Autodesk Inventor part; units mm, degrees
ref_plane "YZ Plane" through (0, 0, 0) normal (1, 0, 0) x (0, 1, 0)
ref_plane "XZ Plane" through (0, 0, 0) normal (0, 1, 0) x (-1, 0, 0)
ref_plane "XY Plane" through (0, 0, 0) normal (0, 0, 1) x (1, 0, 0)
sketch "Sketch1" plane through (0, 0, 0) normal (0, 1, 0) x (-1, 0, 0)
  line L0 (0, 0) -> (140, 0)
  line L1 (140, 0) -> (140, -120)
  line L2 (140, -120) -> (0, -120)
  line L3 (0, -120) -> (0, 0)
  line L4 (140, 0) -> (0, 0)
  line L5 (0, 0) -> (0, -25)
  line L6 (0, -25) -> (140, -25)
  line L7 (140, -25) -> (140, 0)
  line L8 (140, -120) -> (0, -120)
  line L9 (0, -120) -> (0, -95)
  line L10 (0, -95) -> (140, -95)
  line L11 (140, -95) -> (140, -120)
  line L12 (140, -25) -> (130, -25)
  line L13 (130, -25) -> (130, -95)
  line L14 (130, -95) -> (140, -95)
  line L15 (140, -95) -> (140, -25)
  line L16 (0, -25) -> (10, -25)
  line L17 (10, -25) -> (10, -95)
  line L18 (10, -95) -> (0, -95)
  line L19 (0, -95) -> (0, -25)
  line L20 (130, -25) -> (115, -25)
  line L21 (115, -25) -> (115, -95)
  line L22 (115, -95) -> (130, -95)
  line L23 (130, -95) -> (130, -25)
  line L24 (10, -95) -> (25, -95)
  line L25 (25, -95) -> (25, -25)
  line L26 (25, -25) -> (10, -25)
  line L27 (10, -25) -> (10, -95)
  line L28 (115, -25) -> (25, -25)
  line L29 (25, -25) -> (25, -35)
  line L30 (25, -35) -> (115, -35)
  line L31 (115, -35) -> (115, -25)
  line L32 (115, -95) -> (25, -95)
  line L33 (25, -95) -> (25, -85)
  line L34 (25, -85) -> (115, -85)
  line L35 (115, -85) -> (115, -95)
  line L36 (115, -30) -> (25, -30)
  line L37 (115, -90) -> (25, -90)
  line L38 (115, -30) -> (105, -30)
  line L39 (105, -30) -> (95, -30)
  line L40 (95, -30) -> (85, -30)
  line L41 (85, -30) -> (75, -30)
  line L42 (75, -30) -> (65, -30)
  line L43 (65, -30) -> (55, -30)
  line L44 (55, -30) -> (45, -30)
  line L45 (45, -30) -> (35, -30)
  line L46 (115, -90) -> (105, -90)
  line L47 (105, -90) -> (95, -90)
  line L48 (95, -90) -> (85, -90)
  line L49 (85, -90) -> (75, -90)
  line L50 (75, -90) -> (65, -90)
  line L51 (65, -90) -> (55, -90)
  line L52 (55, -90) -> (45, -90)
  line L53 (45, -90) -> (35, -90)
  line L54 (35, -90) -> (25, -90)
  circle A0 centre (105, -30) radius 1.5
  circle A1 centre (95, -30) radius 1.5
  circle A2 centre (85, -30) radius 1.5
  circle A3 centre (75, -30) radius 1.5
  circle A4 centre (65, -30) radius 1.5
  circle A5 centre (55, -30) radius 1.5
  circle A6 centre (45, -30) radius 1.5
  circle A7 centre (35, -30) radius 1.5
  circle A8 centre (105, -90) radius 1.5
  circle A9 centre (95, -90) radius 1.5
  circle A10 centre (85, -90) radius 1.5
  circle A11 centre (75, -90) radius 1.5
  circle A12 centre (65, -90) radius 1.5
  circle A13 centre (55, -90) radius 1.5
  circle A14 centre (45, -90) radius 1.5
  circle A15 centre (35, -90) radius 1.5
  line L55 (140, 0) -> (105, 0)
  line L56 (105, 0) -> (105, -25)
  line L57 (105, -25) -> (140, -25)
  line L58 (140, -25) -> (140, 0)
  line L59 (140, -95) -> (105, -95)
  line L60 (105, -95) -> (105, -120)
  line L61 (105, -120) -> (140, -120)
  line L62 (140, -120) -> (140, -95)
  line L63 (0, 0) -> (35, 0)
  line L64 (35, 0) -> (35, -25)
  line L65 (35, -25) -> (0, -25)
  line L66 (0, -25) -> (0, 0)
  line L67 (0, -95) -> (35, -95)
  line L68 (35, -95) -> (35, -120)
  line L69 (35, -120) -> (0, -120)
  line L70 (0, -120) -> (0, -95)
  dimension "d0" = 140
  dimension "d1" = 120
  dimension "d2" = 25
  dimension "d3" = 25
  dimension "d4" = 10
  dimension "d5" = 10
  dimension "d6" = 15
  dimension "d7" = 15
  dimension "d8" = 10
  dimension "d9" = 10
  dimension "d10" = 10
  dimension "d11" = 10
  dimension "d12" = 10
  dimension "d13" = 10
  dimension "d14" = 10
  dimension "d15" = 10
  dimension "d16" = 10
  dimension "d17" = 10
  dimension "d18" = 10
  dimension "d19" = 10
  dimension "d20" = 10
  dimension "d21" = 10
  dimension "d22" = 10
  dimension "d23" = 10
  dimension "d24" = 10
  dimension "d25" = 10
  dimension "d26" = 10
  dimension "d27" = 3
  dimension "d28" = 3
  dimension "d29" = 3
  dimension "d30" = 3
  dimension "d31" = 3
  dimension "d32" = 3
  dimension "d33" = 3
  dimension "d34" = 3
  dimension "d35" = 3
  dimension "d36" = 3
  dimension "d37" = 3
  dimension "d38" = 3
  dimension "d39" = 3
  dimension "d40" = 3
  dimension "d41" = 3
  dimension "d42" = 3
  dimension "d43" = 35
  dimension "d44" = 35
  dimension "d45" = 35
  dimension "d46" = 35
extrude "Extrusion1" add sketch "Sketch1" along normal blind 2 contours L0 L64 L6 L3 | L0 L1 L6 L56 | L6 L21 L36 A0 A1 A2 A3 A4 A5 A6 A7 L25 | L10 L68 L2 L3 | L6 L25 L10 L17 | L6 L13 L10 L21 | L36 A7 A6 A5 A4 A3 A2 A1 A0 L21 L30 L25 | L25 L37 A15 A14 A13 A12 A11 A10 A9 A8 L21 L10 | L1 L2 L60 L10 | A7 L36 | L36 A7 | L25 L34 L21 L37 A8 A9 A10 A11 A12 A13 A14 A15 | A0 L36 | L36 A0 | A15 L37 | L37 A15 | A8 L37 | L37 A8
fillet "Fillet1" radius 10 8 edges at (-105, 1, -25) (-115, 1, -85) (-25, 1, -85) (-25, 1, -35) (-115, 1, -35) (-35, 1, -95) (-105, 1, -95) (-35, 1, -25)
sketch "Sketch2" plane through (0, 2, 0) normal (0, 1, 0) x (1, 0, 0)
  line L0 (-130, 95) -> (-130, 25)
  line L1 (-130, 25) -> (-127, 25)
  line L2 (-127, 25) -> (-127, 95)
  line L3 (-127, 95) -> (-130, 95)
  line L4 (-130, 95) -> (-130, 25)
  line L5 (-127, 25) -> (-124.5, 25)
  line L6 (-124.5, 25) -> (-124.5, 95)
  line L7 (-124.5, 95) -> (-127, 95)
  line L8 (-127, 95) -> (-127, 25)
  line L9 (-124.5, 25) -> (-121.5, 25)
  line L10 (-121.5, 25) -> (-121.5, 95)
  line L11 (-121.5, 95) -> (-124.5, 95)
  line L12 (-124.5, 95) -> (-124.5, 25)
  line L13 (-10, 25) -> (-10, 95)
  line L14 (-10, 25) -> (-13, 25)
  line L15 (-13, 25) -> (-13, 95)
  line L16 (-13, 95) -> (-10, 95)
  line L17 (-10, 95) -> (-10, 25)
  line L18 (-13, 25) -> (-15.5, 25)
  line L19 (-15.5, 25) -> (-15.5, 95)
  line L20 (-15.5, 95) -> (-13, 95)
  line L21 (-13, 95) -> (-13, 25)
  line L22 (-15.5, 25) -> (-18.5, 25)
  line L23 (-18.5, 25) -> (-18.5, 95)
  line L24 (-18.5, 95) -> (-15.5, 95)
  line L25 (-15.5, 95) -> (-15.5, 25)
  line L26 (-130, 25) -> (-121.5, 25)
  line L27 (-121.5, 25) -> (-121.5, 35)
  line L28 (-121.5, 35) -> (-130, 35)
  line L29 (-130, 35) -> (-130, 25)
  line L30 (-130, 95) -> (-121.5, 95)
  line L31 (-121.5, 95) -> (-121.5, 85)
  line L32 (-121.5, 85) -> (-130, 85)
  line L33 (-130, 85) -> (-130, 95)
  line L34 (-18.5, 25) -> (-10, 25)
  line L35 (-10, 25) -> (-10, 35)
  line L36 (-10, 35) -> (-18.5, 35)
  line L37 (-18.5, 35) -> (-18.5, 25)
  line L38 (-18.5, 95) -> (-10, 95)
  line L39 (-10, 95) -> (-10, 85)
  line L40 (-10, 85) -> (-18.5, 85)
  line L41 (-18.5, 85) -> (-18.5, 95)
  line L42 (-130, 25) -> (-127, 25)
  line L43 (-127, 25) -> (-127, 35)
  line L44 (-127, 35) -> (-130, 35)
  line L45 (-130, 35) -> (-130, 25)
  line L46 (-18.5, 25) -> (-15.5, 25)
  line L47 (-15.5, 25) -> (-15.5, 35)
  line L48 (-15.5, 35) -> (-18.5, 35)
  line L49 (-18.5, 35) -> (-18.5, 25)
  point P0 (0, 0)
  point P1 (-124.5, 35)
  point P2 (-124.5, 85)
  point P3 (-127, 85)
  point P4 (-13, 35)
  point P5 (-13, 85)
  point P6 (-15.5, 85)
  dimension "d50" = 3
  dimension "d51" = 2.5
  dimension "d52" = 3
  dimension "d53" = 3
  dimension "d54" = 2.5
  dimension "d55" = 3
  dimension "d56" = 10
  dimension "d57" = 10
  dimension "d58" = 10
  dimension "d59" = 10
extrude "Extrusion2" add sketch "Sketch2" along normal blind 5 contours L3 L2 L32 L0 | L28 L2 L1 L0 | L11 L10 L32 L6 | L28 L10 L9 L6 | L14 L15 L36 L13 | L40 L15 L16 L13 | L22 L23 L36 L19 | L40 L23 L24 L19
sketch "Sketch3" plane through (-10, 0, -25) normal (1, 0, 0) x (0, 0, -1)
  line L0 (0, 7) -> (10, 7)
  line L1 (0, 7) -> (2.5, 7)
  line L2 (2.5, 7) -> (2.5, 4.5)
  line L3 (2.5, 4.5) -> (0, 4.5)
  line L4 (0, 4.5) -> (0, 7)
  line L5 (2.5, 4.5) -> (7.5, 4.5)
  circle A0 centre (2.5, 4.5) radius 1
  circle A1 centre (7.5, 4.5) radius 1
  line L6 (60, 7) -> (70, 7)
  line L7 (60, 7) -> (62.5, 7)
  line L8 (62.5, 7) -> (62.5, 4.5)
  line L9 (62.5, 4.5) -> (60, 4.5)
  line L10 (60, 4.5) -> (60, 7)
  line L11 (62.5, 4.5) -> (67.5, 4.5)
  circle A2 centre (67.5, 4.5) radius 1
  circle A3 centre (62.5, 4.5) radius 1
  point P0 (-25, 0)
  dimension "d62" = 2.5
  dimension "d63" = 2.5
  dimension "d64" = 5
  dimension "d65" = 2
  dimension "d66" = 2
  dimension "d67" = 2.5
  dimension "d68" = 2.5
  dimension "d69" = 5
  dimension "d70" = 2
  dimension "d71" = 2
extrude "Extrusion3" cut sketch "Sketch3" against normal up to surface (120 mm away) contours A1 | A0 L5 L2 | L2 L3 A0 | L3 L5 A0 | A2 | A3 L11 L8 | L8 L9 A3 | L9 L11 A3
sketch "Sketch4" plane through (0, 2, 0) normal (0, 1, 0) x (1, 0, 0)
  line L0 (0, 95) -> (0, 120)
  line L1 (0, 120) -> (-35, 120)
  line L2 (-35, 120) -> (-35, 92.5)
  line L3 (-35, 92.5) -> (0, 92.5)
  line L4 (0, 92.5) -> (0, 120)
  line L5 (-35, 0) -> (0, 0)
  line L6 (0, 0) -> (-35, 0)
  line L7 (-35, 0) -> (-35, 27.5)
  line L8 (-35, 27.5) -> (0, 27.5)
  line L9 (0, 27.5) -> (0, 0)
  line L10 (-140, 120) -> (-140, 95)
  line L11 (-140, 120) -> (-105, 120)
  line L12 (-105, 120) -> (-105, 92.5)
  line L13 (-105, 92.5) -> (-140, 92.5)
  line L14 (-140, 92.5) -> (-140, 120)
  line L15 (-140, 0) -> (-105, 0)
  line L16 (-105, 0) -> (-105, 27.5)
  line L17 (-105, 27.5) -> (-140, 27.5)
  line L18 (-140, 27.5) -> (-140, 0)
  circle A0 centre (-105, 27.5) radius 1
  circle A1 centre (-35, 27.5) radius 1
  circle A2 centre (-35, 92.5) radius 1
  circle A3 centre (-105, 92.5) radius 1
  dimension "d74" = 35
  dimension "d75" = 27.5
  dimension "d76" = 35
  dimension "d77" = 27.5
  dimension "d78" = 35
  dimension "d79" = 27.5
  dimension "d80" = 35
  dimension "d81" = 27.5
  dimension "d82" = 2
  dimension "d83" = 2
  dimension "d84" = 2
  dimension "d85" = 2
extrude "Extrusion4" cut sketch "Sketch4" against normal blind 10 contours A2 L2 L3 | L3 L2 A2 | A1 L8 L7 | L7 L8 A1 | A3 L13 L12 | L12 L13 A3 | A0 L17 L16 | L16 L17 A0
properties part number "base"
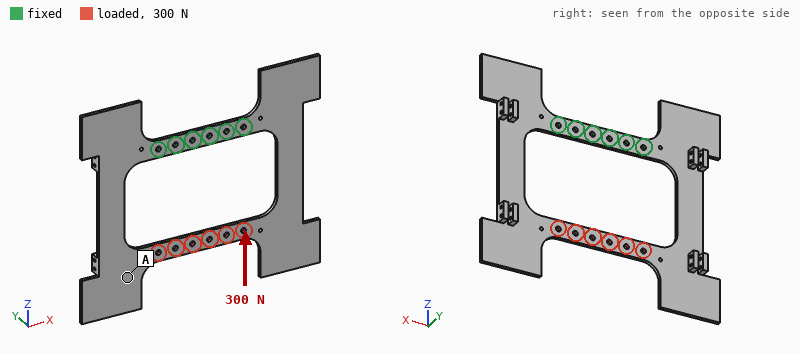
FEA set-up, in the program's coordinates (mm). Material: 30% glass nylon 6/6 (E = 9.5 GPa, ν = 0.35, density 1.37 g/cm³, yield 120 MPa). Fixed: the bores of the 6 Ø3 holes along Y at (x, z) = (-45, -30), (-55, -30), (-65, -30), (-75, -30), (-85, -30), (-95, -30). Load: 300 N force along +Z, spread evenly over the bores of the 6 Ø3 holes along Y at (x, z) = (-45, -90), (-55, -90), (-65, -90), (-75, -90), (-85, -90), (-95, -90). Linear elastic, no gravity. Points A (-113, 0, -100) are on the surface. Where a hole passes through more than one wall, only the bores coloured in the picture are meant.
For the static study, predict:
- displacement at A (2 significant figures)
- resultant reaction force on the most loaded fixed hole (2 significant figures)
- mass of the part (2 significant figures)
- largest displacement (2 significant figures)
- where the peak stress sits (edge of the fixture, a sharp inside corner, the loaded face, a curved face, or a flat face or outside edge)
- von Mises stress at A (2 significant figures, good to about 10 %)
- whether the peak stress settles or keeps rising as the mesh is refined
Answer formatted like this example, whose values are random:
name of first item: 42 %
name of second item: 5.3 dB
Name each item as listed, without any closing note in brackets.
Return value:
displacement at A: 0.53 mm
resultant reaction force on the most loaded fixed hole: 250 N
mass of the part: 22 g
largest displacement: 1.2 mm
where the peak stress sits: edge of the fixture
von Mises stress at A: 8.1 MPa
whether the peak stress settles or keeps rising as the mesh is refined: keeps rising
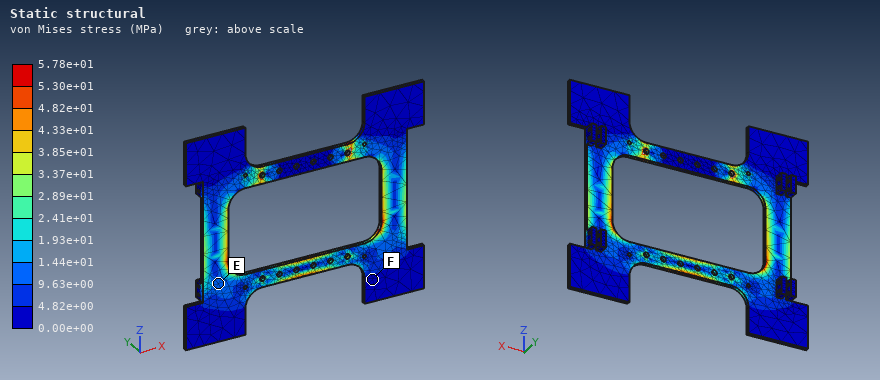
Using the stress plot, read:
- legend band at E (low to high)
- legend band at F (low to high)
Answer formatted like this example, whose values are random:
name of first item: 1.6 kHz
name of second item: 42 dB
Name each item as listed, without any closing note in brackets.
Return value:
legend band at E: 9.63e+00 to 1.44e+01 MPa
legend band at F: 0.00e+00 to 4.82e+00 MPa
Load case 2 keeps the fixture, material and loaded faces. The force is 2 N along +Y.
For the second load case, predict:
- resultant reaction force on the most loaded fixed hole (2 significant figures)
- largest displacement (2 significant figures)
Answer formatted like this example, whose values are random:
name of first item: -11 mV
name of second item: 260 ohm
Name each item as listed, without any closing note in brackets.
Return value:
resultant reaction force on the most loaded fixed hole: 0.99 N
largest displacement: 2.1 mm
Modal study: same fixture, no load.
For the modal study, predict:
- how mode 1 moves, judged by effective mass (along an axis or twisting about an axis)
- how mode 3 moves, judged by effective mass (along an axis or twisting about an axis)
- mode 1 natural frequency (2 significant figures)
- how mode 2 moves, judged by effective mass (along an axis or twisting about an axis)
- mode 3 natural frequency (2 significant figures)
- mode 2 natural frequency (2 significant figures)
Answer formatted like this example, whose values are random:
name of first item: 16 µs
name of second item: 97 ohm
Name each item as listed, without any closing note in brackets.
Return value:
how mode 1 moves, judged by effective mass: along Y
how mode 3 moves, judged by effective mass: along Y
mode 1 natural frequency: 53 Hz
how mode 2 moves, judged by effective mass: twisting about Z
mode 3 natural frequency: 230 Hz
mode 2 natural frequency: 83 Hz
